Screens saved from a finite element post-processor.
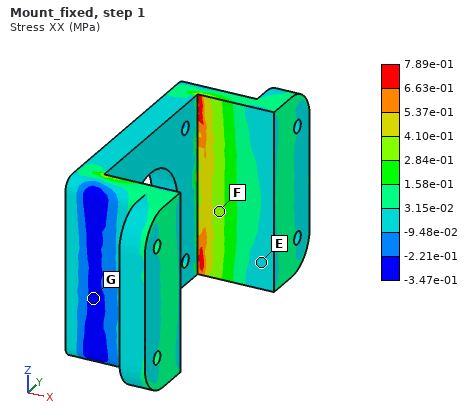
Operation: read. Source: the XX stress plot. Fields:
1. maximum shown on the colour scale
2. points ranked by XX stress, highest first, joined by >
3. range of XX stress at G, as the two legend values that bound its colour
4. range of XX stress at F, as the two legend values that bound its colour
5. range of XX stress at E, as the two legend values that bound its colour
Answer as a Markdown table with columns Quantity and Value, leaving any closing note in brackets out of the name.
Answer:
| Quantity | Value |
|---|---|
| maximum shown on the colour scale | 7.89e-01 MPa |
| points ranked by XX stress, highest first, joined by > | F > E > G |
| range of XX stress at G, as the two legend values that bound its colour | -3.47e-01 to -2.21e-01 MPa |
| range of XX stress at F, as the two legend values that bound its colour | 2.84e-01 to 4.10e-01 MPa |
| range of XX stress at E, as the two legend values that bound its colour | -9.48e-02 to 3.15e-02 MPa |
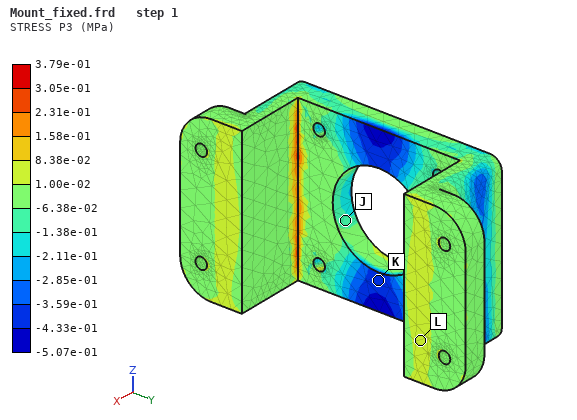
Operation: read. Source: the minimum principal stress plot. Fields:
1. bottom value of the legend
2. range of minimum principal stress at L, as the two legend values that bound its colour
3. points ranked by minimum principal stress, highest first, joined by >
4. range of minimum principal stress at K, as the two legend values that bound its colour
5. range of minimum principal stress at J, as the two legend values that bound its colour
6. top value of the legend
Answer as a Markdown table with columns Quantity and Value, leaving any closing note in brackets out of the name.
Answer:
| Quantity | Value |
|---|---|
| bottom value of the legend | -5.07e-01 MPa |
| range of minimum principal stress at L, as the two legend values that bound its colour | 1.00e-02 to 8.38e-02 MPa |
| points ranked by minimum principal stress, highest first, joined by > | L > J > K |
| range of minimum principal stress at K, as the two legend values that bound its colour | -4.33e-01 to -3.59e-01 MPa |
| range of minimum principal stress at J, as the two legend values that bound its colour | -1.38e-01 to -6.38e-02 MPa |
| top value of the legend | 3.79e-01 MPa |
